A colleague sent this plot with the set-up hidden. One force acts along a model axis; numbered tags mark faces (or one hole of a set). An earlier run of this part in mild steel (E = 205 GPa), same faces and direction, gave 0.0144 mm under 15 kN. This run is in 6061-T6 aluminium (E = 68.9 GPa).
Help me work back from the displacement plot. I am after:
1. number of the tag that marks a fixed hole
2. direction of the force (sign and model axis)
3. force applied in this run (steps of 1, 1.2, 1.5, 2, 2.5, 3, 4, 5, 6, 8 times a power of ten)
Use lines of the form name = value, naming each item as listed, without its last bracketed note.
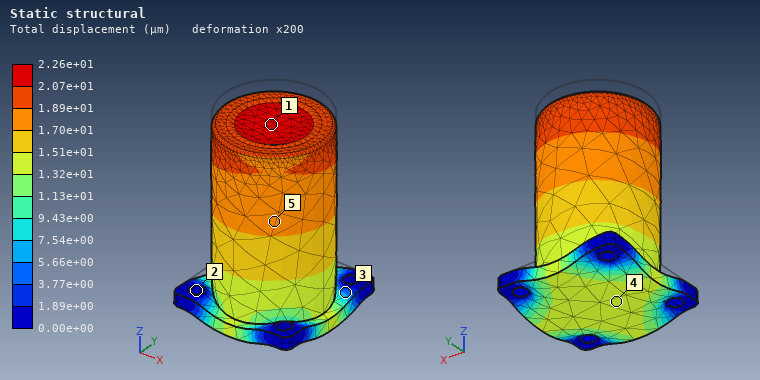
number of the tag that marks a fixed hole = 2
direction of the force = -Z
force applied in this run = 8 kN
